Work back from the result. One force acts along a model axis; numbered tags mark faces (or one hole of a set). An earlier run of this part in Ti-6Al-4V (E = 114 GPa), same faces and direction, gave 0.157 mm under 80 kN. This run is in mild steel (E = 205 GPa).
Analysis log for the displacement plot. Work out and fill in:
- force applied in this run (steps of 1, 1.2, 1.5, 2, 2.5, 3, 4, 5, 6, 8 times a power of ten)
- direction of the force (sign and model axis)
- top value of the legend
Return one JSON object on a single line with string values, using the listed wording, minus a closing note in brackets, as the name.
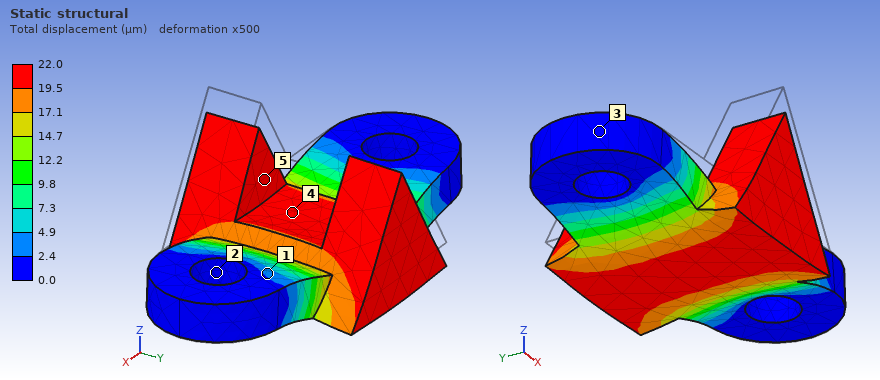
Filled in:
{"force applied in this run": "20 kN", "direction of the force": "-Z", "top value of the legend": "22.0 µm"}
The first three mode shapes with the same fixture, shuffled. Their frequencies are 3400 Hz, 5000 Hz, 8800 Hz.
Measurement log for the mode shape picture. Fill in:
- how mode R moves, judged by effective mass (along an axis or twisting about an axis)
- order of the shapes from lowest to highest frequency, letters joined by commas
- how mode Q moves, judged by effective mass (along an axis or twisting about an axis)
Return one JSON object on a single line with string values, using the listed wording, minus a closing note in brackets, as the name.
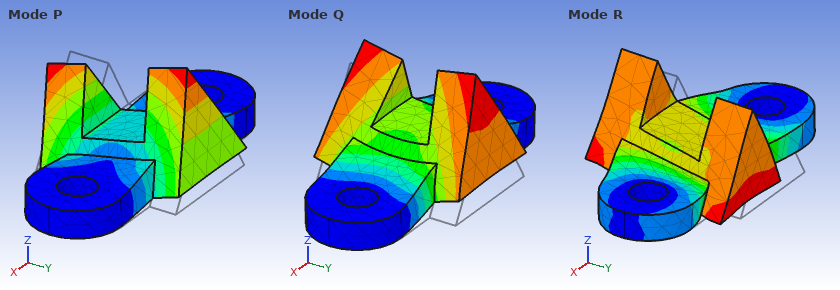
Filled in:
{"how mode R moves, judged by effective mass": "along Y", "order of the shapes from lowest to highest frequency, letters joined by commas": "P, Q, R", "how mode Q moves, judged by effective mass": "along Z"}
